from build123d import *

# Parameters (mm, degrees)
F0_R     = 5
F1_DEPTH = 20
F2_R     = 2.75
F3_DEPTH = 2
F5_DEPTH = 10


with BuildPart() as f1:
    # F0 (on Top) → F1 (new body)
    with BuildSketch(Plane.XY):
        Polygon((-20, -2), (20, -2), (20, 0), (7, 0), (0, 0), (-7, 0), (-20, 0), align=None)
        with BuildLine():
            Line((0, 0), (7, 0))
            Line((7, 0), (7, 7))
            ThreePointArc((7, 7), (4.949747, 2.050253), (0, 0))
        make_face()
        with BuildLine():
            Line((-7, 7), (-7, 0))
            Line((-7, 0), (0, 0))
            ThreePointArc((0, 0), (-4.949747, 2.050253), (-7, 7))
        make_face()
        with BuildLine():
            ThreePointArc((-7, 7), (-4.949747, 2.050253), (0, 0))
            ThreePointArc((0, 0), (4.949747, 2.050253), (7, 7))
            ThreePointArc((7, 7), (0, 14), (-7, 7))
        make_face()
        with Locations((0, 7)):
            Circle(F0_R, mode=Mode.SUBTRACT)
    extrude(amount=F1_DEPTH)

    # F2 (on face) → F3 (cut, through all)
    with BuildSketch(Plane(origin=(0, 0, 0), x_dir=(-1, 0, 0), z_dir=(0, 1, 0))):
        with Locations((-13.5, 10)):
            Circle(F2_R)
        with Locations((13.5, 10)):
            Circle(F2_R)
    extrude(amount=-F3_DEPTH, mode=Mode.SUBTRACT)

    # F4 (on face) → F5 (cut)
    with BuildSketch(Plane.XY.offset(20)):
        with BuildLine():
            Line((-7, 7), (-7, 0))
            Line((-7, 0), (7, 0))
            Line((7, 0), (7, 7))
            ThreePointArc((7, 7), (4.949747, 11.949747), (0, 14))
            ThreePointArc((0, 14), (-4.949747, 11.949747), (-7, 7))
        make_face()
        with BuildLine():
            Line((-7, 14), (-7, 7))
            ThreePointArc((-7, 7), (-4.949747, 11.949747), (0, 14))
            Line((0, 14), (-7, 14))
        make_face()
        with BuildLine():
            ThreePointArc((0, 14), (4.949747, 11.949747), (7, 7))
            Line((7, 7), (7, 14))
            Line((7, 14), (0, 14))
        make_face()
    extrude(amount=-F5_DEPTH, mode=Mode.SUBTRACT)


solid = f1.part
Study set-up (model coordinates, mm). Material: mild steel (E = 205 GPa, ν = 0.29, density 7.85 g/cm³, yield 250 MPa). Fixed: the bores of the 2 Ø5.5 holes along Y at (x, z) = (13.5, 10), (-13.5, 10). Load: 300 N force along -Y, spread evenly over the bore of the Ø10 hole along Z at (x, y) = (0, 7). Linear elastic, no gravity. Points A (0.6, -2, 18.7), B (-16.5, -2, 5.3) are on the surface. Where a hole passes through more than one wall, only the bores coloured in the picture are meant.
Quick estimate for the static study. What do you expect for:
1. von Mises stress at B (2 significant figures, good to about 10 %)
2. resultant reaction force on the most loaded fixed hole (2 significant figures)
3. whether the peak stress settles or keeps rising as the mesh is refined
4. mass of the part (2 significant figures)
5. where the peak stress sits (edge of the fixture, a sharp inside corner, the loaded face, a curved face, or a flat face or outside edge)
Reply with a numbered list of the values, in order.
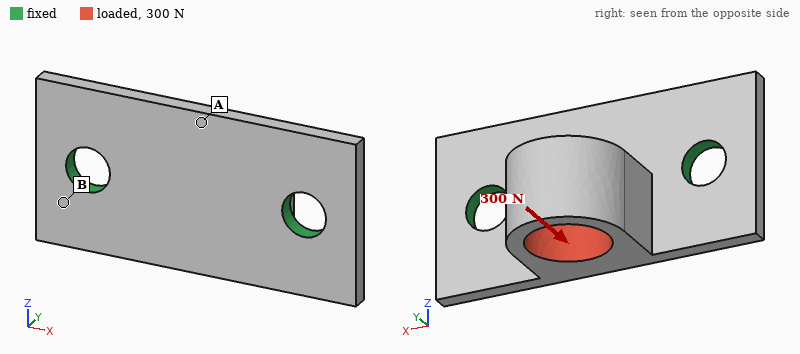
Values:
1. 23 MPa
2. 170 N
3. keeps rising
4. 19 g
5. edge of the fixture
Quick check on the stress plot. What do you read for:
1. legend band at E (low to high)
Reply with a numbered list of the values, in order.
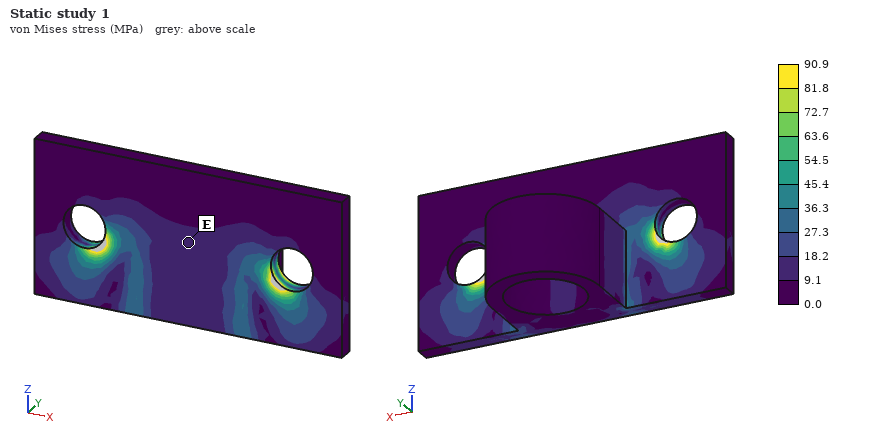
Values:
1. 9.1 to 18.2 MPa
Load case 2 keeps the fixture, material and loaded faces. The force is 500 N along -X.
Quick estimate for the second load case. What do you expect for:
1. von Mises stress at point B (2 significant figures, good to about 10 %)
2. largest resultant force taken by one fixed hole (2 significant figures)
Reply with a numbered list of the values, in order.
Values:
1. 15 MPa
2. 340 N
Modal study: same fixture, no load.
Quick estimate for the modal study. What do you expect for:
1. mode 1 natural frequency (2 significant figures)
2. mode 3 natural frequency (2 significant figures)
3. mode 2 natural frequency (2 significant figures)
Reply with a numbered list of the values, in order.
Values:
1. 6800 Hz
2. 15 kHz
3. 15 kHz
